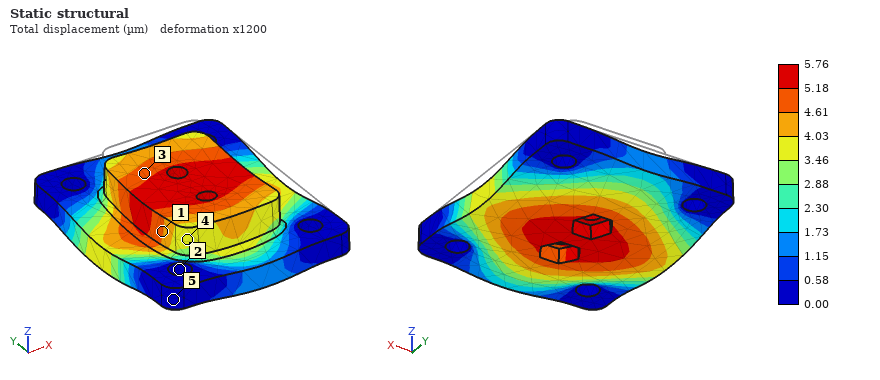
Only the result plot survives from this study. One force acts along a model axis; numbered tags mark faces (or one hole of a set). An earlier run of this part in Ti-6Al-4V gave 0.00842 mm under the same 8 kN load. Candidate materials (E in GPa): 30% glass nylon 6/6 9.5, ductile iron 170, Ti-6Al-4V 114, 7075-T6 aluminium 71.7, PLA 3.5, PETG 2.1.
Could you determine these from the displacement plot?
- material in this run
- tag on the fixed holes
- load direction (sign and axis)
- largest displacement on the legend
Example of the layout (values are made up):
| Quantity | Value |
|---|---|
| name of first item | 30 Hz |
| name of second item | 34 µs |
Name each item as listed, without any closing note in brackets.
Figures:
| Quantity | Value |
|---|---|
| material in this run | ductile iron |
| tag on the fixed holes | 2 |
| load direction | -Z |
| largest displacement on the legend | 5.76 µm |
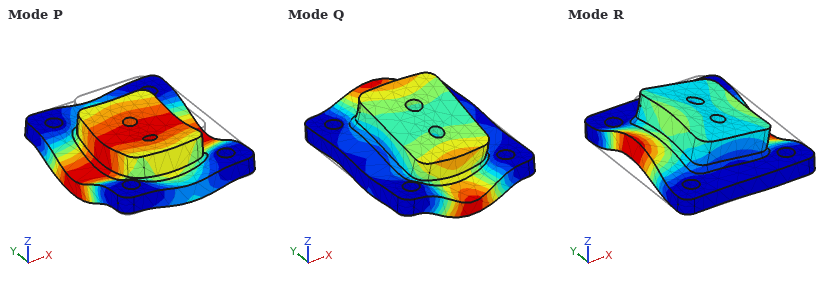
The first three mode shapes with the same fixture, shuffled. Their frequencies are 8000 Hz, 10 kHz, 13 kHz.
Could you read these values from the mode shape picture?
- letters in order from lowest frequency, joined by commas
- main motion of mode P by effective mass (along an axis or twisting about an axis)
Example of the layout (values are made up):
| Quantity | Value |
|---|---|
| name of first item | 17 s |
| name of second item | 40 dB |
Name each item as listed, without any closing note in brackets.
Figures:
| Quantity | Value |
|---|---|
| letters in order from lowest frequency, joined by commas | P, R, Q |
| main motion of mode P by effective mass | along Z |
